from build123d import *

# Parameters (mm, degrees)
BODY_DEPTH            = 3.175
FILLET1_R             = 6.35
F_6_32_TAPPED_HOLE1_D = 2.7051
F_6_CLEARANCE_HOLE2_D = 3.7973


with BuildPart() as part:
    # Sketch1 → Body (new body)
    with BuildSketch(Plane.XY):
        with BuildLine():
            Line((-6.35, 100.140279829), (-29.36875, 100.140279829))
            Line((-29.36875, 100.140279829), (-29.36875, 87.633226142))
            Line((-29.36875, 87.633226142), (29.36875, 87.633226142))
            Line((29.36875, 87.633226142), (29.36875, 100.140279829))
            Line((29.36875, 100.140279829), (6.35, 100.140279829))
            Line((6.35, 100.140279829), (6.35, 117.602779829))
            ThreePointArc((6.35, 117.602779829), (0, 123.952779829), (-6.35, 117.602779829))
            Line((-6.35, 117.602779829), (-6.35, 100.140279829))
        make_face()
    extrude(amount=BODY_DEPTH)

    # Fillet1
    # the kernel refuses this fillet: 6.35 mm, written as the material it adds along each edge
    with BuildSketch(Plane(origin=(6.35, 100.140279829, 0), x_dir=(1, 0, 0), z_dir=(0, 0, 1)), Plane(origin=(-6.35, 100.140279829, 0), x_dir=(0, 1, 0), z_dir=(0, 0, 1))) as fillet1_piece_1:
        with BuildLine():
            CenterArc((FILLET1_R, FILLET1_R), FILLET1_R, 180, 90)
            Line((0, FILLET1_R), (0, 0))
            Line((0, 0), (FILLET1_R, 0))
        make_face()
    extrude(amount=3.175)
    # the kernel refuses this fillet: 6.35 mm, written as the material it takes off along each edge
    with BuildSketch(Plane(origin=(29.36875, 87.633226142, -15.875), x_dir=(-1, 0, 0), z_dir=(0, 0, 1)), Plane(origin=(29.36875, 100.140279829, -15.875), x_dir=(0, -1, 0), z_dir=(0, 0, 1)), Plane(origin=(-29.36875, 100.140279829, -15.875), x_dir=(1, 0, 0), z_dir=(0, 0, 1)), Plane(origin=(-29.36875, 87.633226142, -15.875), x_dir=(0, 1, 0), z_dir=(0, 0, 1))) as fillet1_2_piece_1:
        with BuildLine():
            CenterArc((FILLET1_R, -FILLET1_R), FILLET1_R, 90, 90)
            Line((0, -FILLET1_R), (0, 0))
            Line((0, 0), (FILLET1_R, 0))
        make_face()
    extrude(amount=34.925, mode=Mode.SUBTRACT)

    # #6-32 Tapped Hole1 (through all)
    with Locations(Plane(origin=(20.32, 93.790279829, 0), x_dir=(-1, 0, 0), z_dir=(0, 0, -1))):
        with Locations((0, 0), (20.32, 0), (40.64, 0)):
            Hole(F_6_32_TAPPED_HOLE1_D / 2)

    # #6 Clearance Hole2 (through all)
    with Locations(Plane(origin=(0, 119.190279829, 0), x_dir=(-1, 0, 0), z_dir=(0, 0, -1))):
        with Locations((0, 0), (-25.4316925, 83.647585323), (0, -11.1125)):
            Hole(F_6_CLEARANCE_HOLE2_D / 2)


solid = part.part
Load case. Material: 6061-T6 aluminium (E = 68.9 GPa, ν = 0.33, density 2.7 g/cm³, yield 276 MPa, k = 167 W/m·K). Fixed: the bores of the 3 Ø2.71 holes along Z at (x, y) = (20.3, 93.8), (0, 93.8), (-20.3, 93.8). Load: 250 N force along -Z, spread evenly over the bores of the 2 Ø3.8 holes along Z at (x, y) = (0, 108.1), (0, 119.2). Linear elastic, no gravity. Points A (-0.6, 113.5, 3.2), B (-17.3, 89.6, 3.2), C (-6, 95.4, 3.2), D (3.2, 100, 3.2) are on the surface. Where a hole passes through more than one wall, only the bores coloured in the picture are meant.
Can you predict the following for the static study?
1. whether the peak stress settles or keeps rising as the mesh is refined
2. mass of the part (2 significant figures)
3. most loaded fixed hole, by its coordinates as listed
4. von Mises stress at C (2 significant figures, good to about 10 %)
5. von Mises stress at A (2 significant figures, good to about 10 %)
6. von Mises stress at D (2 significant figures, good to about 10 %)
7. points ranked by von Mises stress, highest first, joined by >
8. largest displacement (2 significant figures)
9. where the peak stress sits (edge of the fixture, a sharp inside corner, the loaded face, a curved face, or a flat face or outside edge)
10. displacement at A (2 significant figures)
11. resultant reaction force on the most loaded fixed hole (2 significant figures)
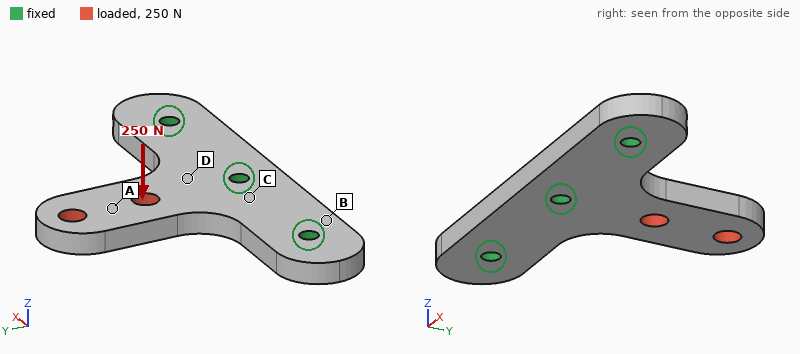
keeps rising
8.3 g
(0, 93.8)
62 MPa
36 MPa
110 MPa
D > C > A > B
0.41 mm
edge of the fixture
0.21 mm
270 N
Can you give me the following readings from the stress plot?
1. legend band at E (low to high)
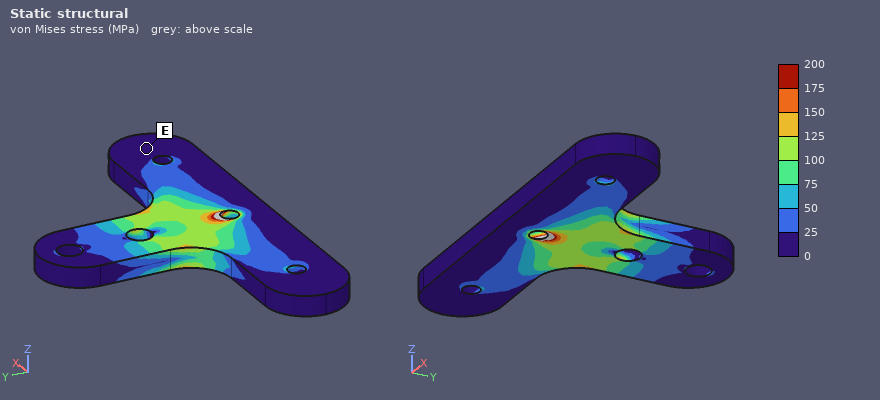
0 to 25 MPa
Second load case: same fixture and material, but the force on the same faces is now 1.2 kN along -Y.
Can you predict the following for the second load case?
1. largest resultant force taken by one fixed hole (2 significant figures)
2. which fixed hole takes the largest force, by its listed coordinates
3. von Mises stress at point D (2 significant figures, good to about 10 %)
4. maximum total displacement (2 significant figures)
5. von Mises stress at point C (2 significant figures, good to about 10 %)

980 N
(0, 93.8)
23 MPa
11 µm
8.3 MPa
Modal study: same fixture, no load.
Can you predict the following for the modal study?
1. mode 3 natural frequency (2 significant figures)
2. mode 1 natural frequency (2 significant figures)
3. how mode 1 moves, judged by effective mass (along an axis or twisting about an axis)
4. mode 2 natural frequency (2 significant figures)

15 kHz
3700 Hz
along Z
15 kHz
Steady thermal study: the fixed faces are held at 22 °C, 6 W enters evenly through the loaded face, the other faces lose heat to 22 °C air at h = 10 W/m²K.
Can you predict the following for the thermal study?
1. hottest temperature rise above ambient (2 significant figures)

18 K
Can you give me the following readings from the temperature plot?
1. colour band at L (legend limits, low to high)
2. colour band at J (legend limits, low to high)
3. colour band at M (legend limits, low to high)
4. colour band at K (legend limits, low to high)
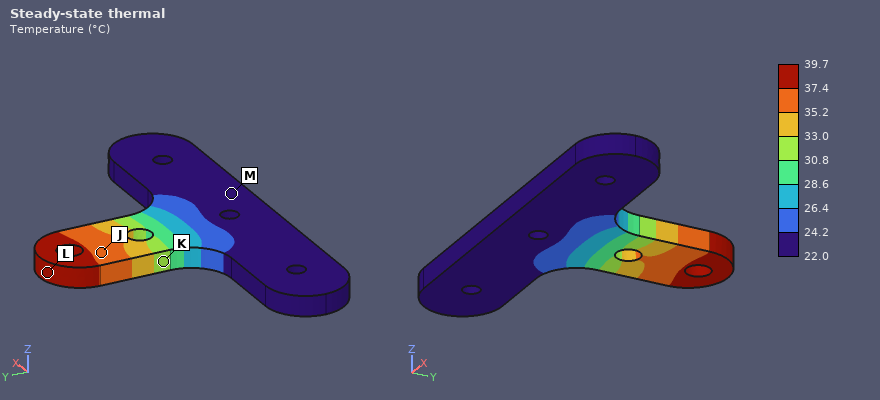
37.4 to 39.7 °C
35.2 to 37.4 °C
22.0 to 24.2 °C
30.8 to 33.0 °C
